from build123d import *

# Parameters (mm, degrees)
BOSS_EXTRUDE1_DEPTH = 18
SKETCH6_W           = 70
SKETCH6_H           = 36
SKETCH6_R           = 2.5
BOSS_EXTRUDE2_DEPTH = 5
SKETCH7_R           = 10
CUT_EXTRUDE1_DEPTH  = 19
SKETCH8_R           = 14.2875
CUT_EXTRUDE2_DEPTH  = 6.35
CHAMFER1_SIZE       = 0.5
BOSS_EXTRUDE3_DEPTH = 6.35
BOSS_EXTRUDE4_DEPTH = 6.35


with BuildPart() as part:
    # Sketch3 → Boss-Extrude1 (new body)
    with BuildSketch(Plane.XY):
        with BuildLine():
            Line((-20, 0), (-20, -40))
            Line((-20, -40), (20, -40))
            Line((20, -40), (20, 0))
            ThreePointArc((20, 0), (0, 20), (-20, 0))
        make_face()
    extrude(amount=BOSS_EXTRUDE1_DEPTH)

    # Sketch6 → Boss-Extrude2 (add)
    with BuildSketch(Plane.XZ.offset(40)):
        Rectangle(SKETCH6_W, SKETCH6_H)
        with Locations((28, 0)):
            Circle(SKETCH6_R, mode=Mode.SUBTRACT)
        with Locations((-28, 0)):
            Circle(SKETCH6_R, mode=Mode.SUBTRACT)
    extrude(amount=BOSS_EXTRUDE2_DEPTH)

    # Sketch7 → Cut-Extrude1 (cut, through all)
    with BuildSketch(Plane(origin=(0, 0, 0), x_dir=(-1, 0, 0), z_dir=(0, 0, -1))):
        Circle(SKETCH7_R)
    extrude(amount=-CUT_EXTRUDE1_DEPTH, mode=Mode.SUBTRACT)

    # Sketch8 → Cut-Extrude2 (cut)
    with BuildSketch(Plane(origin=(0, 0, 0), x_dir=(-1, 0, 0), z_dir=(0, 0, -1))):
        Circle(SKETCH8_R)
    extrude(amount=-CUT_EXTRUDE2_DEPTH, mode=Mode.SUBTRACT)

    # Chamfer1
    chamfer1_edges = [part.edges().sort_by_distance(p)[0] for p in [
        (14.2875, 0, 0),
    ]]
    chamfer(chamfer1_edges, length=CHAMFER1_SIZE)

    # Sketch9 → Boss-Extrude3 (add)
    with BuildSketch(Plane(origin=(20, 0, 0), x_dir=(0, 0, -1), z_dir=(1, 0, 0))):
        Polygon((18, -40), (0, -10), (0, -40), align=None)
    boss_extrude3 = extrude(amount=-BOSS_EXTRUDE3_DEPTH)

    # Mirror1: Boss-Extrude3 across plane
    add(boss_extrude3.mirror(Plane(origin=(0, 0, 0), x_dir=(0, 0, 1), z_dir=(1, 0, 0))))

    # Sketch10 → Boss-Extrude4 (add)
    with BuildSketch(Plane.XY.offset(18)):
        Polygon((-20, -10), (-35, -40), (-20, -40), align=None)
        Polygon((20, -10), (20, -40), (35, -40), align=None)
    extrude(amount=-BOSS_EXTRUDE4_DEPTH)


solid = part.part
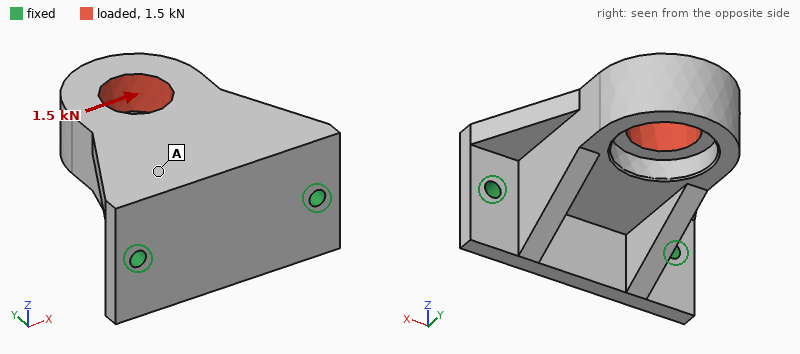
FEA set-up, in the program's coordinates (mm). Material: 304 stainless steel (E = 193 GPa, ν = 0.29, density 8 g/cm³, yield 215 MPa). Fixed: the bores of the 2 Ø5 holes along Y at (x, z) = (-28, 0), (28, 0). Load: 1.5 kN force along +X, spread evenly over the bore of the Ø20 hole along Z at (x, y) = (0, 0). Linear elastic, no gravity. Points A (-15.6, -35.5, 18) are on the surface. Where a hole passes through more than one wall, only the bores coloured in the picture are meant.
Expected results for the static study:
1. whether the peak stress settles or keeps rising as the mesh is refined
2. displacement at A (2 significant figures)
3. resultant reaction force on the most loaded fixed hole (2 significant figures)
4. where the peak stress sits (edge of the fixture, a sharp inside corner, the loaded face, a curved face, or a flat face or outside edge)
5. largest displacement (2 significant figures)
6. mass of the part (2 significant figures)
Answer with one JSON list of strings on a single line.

["keeps rising", "3.4 µm", "1.5 kN", "edge of the fixture", "16 µm", "410 g"]
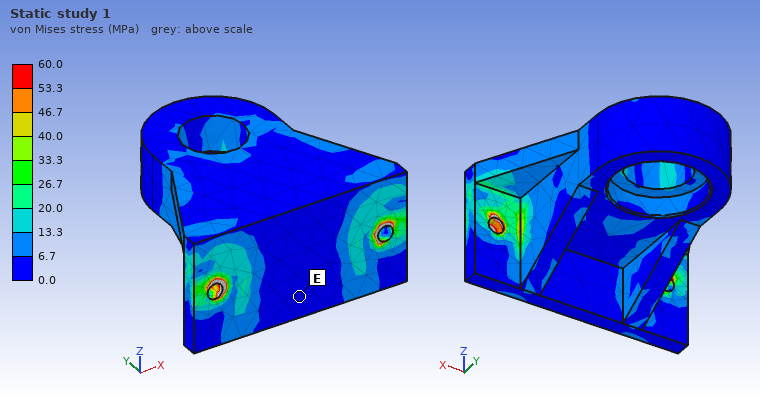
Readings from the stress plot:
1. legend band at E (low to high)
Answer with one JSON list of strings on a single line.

["0.0 to 6.7 MPa"]
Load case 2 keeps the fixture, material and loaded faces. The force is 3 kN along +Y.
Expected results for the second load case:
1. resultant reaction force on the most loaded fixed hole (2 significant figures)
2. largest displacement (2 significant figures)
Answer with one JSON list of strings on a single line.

["1.6 kN", "90 µm"]
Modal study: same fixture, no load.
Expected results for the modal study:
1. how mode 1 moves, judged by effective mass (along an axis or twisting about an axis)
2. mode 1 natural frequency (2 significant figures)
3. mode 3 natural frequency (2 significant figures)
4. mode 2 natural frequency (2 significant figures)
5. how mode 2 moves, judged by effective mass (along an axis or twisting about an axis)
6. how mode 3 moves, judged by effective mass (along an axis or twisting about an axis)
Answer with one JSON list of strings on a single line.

["along Z", "1400 Hz", "6200 Hz", "4500 Hz", "along X", "along Y"]
